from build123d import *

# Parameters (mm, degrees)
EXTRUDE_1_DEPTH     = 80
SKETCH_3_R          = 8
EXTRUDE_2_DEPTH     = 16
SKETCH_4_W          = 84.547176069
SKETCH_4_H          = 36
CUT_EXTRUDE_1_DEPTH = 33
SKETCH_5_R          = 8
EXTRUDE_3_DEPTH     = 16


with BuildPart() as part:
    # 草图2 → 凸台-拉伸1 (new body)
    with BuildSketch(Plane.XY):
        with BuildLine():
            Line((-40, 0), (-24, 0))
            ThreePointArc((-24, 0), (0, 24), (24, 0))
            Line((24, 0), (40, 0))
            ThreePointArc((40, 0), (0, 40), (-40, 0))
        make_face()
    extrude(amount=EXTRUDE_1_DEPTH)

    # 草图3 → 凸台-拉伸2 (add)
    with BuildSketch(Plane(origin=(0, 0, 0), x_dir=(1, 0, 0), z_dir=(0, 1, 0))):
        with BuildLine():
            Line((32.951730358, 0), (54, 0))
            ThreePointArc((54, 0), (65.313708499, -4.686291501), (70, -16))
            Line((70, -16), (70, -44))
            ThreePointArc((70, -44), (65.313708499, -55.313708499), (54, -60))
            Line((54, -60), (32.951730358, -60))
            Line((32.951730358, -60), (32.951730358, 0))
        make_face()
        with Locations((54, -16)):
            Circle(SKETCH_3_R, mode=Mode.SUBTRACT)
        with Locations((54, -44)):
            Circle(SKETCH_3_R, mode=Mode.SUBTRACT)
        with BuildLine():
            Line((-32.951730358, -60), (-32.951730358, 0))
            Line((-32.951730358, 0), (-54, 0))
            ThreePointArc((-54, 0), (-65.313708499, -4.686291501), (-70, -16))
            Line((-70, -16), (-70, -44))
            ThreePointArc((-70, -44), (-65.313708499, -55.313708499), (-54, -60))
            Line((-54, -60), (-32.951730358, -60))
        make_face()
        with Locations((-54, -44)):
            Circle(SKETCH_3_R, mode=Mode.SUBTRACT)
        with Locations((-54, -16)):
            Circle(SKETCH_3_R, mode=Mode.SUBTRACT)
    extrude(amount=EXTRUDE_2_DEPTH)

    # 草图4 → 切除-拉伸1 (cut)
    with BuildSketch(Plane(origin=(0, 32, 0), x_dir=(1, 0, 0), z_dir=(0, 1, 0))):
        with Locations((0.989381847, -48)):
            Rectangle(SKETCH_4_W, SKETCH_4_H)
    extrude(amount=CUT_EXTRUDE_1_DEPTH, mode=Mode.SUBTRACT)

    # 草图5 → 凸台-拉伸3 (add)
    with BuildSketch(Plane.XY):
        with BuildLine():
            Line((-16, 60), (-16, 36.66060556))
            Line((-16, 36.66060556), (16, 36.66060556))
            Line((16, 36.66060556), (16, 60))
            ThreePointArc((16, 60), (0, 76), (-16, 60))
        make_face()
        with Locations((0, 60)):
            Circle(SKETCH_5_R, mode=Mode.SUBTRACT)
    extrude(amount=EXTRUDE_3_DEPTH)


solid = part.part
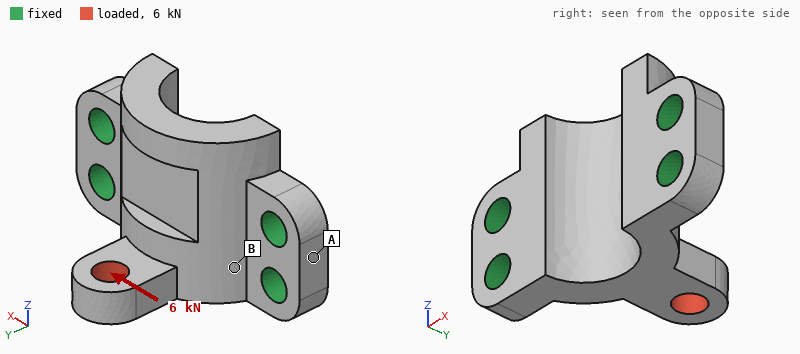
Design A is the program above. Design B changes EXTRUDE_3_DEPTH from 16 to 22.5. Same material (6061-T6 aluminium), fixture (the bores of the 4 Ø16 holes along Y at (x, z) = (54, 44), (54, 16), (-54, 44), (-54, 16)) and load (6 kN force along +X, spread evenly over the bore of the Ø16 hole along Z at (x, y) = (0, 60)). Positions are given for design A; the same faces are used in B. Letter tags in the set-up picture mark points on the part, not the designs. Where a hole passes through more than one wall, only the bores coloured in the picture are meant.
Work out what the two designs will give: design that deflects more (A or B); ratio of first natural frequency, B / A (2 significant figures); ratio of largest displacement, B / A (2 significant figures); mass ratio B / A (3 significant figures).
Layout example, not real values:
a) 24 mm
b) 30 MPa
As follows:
a) A
b) 0.97
c) 0.77
d) 1.03
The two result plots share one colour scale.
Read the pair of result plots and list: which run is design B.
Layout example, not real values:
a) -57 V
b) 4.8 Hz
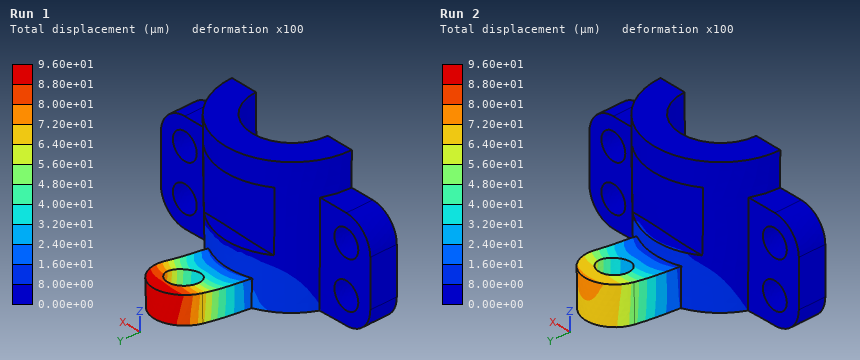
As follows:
a) Run 2
